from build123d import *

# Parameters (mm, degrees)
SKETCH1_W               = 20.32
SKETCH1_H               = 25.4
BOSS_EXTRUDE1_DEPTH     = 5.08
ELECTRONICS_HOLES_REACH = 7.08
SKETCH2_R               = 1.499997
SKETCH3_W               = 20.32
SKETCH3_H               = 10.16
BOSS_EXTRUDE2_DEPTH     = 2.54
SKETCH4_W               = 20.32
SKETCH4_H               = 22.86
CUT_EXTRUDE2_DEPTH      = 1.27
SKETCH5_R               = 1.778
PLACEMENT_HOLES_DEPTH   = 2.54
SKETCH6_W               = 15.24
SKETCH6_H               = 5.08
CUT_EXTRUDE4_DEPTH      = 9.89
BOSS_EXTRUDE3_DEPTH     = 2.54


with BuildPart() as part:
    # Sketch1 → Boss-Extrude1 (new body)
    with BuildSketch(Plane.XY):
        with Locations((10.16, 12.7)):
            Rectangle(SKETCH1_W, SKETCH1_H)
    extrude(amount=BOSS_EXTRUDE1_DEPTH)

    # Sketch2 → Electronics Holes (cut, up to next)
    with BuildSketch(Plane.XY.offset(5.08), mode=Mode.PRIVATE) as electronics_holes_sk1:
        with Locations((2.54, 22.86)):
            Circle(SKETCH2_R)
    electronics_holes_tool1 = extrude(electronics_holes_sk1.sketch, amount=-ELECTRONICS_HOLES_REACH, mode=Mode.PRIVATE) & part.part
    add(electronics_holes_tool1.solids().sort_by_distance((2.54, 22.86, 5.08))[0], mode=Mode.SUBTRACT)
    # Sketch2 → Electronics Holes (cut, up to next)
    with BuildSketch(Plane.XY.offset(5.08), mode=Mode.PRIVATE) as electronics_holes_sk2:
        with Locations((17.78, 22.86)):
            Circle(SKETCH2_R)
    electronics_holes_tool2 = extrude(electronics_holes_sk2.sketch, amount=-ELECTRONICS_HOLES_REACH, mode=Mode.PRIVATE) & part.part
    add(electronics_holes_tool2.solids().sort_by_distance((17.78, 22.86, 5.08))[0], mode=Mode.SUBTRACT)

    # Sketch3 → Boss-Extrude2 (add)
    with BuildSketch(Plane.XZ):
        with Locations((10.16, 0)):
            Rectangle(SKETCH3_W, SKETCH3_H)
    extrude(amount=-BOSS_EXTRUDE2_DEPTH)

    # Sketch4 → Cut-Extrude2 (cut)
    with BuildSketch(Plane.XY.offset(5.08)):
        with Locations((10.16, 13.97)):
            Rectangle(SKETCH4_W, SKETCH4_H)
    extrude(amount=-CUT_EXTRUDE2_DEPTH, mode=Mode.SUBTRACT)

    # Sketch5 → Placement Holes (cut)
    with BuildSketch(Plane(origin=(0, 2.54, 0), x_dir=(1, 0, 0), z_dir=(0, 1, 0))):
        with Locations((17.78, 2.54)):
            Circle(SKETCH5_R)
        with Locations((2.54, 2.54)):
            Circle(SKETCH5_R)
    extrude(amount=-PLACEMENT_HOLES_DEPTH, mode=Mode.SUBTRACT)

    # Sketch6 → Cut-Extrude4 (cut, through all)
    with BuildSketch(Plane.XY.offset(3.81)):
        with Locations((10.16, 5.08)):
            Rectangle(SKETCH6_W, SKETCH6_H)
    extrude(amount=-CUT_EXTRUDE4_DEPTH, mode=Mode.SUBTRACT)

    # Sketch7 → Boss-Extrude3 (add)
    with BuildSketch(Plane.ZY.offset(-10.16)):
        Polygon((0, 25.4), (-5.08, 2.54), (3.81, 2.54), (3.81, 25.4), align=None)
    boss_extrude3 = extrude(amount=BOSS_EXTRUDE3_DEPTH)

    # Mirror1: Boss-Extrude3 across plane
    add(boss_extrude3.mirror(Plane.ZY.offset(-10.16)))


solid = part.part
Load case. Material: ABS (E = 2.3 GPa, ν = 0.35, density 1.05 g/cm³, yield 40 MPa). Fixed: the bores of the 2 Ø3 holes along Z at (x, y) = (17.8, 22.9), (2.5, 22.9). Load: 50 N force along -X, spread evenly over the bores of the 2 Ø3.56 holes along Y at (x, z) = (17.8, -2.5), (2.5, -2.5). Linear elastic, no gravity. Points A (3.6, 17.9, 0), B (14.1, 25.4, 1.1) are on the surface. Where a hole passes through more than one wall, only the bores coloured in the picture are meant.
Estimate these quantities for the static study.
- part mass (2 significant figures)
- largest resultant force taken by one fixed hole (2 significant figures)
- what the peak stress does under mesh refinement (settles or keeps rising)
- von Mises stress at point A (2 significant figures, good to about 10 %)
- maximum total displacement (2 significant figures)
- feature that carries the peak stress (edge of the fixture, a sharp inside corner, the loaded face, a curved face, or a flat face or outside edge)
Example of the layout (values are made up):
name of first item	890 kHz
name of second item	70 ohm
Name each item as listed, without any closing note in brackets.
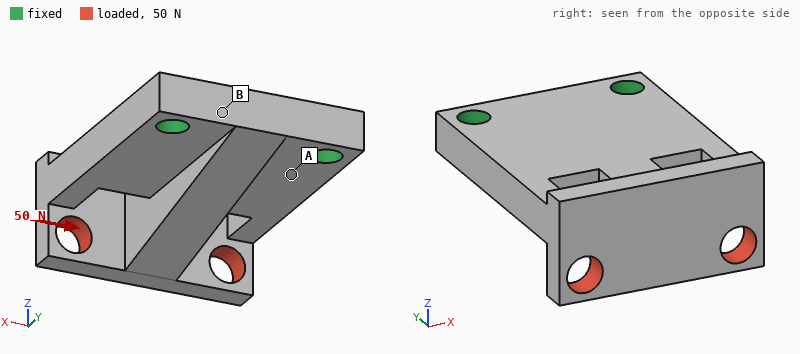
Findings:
part mass	2.4 g
largest resultant force taken by one fixed hole	73 N
what the peak stress does under mesh refinement	keeps rising
von Mises stress at point A	3.2 MPa
maximum total displacement	0.15 mm
feature that carries the peak stress	edge of the fixture
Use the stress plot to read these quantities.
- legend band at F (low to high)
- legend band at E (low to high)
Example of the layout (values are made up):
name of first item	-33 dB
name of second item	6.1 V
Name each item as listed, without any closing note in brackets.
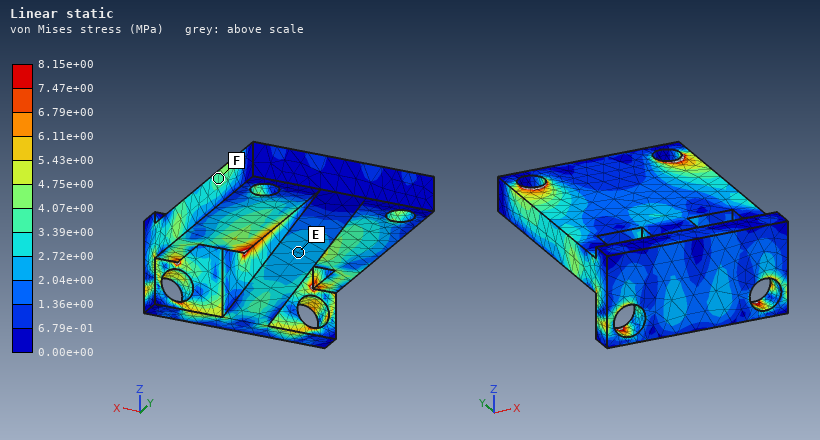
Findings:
legend band at F	3.39e+00 to 4.07e+00 MPa
legend band at E	2.04e+00 to 2.72e+00 MPa
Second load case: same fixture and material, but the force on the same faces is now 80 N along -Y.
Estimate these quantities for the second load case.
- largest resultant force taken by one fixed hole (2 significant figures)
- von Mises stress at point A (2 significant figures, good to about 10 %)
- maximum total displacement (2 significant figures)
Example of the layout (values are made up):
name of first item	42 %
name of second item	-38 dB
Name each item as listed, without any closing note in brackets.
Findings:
largest resultant force taken by one fixed hole	41 N
von Mises stress at point A	6.7 MPa
maximum total displacement	0.41 mm
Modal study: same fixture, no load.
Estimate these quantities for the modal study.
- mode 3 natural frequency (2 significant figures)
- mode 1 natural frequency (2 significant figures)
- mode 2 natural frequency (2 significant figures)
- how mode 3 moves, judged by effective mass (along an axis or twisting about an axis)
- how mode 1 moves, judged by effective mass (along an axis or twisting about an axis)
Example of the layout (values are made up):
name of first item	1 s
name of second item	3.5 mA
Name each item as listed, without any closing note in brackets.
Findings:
mode 3 natural frequency	5200 Hz
mode 1 natural frequency	1500 Hz
mode 2 natural frequency	4000 Hz
how mode 3 moves, judged by effective mass	along X
how mode 1 moves, judged by effective mass	along Z
